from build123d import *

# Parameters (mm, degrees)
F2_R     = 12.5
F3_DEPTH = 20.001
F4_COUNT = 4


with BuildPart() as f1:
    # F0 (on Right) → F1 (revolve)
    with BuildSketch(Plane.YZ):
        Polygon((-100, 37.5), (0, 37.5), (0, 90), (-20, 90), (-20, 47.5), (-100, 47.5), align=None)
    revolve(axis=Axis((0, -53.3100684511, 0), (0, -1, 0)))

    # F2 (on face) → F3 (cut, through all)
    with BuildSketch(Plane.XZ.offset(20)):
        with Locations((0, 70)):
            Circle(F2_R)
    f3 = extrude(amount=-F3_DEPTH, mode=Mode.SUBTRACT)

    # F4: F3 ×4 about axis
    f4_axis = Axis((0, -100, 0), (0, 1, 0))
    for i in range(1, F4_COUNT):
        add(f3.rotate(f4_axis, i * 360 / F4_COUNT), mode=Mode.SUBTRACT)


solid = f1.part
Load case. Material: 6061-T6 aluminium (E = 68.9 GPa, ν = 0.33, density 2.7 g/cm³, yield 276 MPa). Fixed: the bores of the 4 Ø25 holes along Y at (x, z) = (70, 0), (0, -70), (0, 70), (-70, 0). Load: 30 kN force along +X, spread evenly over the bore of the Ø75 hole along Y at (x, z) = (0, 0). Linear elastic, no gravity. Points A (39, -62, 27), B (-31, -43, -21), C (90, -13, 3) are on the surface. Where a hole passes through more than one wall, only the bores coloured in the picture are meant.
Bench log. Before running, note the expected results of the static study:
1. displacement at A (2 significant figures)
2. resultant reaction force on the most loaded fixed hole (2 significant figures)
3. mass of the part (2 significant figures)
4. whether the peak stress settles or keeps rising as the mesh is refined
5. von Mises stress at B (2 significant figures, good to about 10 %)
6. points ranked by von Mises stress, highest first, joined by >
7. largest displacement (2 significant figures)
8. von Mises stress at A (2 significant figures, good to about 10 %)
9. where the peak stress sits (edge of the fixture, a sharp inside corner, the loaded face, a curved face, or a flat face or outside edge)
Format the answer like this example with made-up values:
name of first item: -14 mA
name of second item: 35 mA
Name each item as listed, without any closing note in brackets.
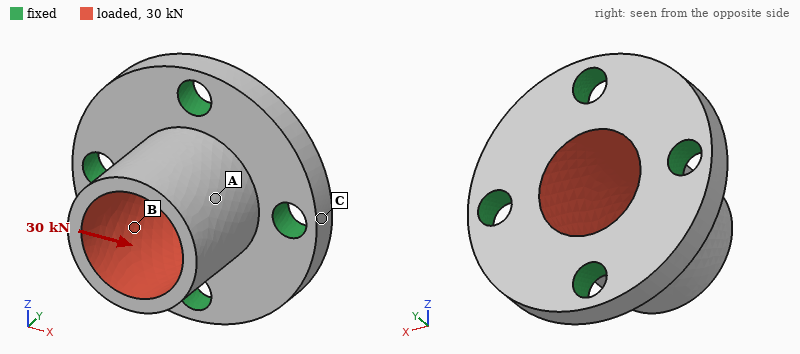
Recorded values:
displacement at A: 44 µm
resultant reaction force on the most loaded fixed hole: 13 kN
mass of the part: 1.6 kg
whether the peak stress settles or keeps rising as the mesh is refined: keeps rising
von Mises stress at B: 19 MPa
points ranked by von Mises stress, highest first, joined by >: B > A > C
largest displacement: 67 µm
von Mises stress at A: 9.1 MPa
where the peak stress sits: edge of the fixture
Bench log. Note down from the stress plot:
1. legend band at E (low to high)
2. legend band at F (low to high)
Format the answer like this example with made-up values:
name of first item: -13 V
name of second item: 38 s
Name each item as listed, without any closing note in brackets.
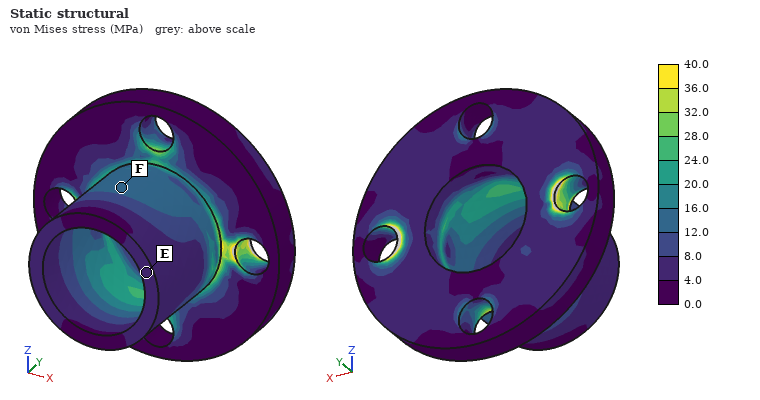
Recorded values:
legend band at E: 4.0 to 8.0 MPa
legend band at F: 12.0 to 16.0 MPa
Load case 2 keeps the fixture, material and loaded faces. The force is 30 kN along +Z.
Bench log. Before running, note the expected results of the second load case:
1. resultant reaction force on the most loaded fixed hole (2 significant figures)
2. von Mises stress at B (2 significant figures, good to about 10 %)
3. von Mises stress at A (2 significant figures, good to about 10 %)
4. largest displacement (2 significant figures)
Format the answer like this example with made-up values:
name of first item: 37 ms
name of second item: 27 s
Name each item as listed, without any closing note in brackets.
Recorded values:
resultant reaction force on the most loaded fixed hole: 13 kN
von Mises stress at B: 22 MPa
von Mises stress at A: 12 MPa
largest displacement: 67 µm
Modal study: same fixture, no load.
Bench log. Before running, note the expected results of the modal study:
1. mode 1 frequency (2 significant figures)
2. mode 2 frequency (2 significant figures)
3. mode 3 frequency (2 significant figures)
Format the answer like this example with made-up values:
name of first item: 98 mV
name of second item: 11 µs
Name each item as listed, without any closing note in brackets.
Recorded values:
mode 1 frequency: 4500 Hz
mode 2 frequency: 4500 Hz
mode 3 frequency: 4600 Hz
